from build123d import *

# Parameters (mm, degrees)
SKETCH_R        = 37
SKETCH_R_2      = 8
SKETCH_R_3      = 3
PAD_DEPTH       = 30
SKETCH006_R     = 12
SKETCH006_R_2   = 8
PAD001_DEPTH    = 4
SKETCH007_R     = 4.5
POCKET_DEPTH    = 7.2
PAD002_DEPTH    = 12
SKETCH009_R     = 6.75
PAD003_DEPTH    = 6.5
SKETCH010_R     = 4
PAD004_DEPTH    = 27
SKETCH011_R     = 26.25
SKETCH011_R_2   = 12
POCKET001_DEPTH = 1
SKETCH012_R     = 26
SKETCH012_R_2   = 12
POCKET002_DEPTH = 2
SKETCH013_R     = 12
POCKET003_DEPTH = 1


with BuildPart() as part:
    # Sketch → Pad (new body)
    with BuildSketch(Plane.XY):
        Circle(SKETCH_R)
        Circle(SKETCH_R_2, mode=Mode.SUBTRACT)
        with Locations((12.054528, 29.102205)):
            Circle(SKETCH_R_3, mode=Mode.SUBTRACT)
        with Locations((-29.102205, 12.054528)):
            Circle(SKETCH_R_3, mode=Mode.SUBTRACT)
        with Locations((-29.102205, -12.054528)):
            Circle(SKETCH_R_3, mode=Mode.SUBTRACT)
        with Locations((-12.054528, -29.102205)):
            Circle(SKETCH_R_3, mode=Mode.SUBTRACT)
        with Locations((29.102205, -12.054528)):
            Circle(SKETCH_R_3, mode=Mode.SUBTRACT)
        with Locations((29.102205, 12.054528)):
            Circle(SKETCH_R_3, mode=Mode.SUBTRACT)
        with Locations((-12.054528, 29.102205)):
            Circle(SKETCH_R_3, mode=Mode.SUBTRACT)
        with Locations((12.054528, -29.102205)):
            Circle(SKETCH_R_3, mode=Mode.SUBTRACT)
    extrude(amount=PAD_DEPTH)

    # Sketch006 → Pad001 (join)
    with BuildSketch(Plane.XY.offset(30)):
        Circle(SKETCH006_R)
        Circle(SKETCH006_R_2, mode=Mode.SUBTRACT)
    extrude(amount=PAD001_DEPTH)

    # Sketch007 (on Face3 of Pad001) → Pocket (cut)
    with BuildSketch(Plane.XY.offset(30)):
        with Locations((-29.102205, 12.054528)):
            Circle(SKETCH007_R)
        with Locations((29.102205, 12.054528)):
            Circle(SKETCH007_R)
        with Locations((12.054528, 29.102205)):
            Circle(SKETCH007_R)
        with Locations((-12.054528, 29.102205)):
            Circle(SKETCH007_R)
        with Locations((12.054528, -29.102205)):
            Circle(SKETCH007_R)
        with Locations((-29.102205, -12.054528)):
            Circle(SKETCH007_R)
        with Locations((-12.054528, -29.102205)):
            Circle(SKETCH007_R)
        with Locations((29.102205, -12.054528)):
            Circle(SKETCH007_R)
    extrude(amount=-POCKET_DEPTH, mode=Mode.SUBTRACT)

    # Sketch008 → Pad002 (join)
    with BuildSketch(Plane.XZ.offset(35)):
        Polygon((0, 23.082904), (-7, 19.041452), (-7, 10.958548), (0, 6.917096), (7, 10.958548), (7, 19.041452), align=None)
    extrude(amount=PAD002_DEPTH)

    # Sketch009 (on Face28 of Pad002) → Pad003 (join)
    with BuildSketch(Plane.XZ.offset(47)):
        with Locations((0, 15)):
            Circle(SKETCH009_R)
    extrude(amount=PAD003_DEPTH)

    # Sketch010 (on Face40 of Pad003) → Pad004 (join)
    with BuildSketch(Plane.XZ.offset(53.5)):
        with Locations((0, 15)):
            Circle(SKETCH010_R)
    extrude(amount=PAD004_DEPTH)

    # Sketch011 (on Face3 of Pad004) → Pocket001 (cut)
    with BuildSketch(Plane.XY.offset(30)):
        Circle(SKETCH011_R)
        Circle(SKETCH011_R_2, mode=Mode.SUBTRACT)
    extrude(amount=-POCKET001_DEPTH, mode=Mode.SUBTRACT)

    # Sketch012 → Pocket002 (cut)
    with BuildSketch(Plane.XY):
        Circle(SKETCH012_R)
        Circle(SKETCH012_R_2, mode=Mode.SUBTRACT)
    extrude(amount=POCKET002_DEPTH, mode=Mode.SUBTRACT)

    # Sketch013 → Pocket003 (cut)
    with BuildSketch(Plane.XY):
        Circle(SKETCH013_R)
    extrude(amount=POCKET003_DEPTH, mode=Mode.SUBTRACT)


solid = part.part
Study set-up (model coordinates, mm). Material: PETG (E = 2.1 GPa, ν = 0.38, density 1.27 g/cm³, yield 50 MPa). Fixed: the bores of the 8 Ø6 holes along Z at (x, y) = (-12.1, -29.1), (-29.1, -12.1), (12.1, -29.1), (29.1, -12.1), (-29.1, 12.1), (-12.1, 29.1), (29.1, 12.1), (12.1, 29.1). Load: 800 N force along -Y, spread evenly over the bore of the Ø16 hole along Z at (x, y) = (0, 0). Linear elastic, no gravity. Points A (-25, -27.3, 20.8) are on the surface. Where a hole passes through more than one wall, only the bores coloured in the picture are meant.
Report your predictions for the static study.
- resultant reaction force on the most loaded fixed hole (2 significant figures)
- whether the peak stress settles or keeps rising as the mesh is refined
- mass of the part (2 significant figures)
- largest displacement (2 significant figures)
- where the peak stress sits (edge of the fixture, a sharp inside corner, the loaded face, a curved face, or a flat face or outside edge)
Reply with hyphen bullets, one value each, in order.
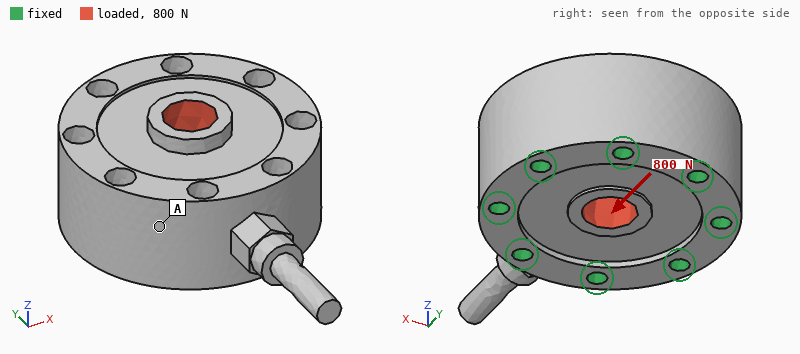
- 160 N
- keeps rising
- 140 g
- 13 µm
- edge of the fixture
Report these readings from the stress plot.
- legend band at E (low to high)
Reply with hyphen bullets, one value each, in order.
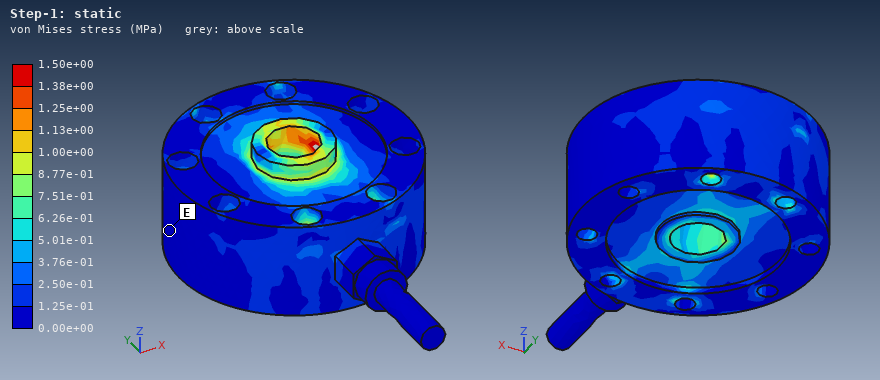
- 0.00e+00 to 1.25e-01 MPa
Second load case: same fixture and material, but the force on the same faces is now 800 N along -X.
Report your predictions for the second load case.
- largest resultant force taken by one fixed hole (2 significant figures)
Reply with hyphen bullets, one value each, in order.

- 160 N
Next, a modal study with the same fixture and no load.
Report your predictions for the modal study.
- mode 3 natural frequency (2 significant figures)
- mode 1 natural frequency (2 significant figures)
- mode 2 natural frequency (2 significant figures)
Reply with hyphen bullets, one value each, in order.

- 4800 Hz
- 1400 Hz
- 1400 Hz
